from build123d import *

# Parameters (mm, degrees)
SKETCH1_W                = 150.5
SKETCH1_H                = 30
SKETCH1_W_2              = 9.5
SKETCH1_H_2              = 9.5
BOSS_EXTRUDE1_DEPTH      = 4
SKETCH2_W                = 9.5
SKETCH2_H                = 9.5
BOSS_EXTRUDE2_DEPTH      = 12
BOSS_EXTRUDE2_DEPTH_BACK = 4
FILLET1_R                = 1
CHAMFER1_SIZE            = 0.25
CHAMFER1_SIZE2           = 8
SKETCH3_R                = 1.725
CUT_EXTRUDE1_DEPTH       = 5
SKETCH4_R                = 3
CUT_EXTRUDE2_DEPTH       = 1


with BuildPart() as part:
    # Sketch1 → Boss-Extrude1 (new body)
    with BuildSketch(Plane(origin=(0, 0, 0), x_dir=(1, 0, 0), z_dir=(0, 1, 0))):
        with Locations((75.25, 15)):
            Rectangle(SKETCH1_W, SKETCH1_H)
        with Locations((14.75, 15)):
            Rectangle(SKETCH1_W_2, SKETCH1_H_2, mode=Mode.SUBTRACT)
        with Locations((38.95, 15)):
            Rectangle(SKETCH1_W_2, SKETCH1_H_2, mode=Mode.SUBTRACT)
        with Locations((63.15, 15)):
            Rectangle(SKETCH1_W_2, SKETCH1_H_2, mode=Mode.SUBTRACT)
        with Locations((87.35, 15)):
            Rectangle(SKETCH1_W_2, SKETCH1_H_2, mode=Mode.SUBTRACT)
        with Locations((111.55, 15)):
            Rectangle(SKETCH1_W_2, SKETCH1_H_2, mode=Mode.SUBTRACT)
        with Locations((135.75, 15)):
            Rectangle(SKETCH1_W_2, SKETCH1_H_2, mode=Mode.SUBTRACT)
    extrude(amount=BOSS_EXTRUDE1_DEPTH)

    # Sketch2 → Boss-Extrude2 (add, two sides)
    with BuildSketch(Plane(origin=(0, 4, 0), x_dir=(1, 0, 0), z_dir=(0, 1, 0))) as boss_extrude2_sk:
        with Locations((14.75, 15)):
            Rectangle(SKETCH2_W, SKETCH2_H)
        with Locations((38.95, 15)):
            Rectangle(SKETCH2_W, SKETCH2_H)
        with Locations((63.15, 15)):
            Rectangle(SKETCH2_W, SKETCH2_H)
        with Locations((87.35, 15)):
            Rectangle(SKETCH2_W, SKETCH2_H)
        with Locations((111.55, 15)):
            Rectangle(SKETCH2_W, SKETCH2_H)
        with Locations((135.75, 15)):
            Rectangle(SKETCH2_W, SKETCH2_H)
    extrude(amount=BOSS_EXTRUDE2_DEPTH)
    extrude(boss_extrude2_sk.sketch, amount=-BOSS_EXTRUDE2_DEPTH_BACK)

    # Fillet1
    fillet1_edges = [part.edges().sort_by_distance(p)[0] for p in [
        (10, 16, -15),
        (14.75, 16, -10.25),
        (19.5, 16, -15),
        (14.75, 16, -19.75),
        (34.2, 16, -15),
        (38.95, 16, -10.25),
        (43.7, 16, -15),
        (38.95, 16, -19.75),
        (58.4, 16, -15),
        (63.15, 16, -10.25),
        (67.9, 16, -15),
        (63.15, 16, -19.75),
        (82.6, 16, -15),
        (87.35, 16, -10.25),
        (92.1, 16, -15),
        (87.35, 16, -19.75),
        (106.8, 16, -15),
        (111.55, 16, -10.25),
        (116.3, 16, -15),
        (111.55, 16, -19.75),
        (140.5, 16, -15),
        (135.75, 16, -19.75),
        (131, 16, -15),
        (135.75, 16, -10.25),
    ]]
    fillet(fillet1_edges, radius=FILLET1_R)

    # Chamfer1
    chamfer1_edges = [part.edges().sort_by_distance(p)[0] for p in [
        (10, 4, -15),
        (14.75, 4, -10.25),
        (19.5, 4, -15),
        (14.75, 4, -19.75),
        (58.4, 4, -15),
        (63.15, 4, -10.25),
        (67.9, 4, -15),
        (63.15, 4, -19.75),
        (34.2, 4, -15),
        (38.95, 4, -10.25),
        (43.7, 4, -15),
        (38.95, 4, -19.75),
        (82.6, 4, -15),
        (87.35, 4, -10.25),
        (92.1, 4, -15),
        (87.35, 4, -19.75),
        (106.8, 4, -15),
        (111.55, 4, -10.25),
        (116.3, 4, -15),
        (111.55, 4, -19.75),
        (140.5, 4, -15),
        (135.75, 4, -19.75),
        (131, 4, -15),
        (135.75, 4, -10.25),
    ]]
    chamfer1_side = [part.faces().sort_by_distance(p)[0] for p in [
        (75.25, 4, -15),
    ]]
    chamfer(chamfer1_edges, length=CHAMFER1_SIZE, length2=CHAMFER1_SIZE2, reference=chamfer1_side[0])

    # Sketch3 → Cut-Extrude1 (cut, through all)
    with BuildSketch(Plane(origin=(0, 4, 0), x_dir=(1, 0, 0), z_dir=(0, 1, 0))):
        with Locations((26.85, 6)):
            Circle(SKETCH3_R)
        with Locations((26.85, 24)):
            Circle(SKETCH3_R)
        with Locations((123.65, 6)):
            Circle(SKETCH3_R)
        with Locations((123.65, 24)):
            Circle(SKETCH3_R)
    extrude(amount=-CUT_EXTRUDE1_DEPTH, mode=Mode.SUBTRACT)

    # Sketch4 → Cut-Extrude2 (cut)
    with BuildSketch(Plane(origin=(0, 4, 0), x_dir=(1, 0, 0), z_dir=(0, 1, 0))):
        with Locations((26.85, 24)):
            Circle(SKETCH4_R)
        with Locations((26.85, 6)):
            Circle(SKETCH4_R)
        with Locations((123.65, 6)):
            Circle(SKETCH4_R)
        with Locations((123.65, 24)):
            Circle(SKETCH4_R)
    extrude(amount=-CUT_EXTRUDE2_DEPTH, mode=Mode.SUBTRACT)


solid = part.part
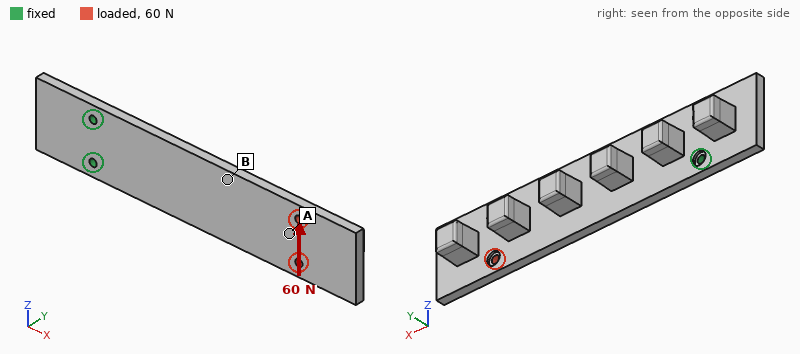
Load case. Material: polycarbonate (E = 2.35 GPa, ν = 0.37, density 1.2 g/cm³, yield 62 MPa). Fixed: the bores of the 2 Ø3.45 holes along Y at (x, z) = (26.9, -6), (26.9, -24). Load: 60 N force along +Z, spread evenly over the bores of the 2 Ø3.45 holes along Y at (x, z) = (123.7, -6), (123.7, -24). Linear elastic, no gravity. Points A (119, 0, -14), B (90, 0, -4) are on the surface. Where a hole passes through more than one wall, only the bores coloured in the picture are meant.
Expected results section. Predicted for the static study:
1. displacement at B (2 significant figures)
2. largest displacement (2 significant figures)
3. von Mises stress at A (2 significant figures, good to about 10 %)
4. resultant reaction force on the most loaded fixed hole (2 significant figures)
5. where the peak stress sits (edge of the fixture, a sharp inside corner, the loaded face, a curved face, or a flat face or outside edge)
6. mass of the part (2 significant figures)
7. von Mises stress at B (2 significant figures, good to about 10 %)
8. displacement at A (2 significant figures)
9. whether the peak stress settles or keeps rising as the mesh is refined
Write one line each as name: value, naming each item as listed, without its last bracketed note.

displacement at B: 0.56 mm
largest displacement: 1.4 mm
von Mises stress at A: 1.4 MPa
resultant reaction force on the most loaded fixed hole: 300 N
where the peak stress sits: edge of the fixture
mass of the part: 29 g
von Mises stress at B: 2.7 MPa
displacement at A: 0.95 mm
whether the peak stress settles or keeps rising as the mesh is refined: keeps rising
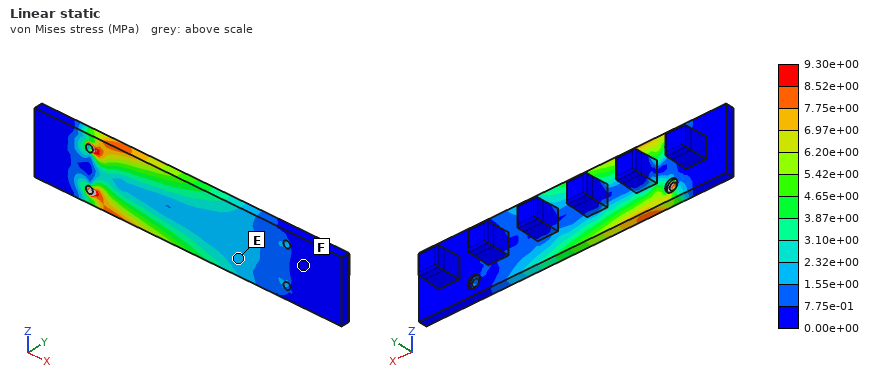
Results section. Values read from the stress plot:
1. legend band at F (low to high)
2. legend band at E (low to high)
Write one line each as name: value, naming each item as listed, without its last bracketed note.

legend band at F: 0.00e+00 to 7.75e-01 MPa
legend band at E: 1.55e+00 to 2.32e+00 MPa
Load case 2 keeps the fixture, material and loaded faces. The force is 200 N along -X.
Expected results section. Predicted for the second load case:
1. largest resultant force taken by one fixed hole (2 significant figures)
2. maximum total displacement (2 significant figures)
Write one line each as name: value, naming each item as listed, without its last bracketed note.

largest resultant force taken by one fixed hole: 100 N
maximum total displacement: 1.8 mm
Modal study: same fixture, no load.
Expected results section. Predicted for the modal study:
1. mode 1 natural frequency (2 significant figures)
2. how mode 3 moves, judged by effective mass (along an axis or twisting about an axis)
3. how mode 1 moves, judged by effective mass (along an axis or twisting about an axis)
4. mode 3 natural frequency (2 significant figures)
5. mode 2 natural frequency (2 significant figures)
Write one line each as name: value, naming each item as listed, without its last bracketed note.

mode 1 natural frequency: 54 Hz
how mode 3 moves, judged by effective mass: along Z
how mode 1 moves, judged by effective mass: along Y
mode 3 natural frequency: 350 Hz
mode 2 natural frequency: 330 Hz
